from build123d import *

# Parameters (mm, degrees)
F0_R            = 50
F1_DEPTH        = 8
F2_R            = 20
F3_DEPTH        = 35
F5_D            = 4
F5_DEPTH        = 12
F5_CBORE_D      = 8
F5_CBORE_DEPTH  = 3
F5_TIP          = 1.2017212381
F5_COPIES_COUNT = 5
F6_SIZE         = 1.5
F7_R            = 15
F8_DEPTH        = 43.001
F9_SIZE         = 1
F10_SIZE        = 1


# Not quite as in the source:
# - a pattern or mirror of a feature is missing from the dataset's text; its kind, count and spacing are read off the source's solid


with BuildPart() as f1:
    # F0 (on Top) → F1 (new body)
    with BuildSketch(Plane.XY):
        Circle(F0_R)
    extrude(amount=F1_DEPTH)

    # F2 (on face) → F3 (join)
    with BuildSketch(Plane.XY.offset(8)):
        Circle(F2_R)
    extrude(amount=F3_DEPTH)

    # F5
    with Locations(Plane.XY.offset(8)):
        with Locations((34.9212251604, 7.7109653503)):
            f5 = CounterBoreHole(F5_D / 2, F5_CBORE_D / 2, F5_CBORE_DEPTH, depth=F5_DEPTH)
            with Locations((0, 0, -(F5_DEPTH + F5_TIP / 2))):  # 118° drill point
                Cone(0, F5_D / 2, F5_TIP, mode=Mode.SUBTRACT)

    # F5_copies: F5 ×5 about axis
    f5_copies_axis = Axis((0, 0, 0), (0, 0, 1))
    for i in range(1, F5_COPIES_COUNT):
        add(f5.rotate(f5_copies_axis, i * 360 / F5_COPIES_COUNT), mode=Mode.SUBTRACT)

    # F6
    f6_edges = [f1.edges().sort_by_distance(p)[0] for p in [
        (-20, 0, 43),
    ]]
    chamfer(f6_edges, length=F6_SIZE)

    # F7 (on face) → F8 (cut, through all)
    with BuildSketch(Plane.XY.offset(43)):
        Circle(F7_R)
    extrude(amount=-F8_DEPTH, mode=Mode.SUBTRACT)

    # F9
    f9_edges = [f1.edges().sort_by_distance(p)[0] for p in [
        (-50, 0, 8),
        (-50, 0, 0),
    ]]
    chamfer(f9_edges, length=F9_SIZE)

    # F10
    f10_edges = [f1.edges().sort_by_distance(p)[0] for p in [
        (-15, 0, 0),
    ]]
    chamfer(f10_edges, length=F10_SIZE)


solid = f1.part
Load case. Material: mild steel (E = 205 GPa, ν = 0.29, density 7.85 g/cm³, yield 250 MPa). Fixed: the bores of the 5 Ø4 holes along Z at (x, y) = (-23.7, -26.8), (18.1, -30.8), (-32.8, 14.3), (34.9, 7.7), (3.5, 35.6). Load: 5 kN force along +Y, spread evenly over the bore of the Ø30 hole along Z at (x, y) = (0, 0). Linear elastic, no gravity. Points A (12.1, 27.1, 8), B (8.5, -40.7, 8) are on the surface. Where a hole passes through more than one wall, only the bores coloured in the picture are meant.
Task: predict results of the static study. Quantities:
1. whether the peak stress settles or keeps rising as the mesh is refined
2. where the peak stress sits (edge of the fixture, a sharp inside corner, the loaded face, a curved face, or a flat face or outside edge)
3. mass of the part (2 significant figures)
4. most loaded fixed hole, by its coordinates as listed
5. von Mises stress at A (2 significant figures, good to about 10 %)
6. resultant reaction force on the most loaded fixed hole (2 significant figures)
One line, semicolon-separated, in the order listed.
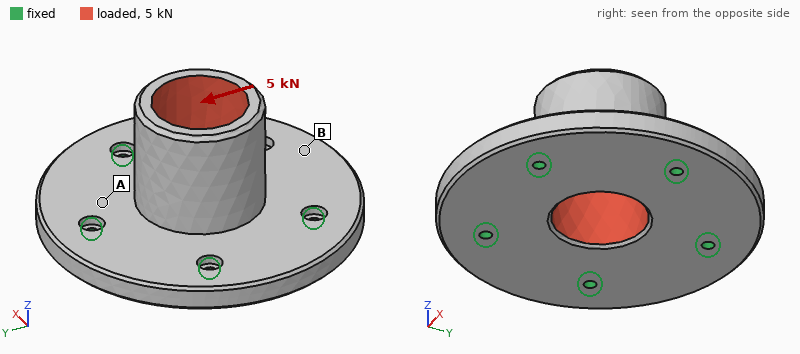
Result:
keeps rising; edge of the fixture; 590 g; (3.5, 35.6); 14 MPa; 1.9 kN
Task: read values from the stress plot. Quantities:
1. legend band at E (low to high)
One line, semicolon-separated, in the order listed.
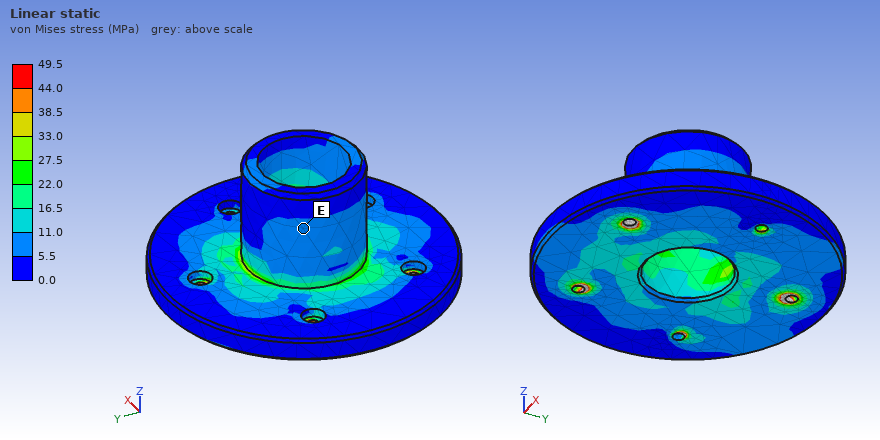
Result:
5.5 to 11.0 MPa
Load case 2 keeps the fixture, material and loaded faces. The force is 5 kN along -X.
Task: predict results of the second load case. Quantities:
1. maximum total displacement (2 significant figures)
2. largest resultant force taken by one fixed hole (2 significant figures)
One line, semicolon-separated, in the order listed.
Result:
16 µm; 1.9 kN
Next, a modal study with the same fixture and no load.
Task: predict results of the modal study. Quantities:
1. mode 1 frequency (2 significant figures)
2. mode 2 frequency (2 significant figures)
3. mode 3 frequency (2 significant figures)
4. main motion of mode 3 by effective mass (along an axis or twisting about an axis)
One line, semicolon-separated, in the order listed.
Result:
7300 Hz; 7300 Hz; 8200 Hz; along Z
